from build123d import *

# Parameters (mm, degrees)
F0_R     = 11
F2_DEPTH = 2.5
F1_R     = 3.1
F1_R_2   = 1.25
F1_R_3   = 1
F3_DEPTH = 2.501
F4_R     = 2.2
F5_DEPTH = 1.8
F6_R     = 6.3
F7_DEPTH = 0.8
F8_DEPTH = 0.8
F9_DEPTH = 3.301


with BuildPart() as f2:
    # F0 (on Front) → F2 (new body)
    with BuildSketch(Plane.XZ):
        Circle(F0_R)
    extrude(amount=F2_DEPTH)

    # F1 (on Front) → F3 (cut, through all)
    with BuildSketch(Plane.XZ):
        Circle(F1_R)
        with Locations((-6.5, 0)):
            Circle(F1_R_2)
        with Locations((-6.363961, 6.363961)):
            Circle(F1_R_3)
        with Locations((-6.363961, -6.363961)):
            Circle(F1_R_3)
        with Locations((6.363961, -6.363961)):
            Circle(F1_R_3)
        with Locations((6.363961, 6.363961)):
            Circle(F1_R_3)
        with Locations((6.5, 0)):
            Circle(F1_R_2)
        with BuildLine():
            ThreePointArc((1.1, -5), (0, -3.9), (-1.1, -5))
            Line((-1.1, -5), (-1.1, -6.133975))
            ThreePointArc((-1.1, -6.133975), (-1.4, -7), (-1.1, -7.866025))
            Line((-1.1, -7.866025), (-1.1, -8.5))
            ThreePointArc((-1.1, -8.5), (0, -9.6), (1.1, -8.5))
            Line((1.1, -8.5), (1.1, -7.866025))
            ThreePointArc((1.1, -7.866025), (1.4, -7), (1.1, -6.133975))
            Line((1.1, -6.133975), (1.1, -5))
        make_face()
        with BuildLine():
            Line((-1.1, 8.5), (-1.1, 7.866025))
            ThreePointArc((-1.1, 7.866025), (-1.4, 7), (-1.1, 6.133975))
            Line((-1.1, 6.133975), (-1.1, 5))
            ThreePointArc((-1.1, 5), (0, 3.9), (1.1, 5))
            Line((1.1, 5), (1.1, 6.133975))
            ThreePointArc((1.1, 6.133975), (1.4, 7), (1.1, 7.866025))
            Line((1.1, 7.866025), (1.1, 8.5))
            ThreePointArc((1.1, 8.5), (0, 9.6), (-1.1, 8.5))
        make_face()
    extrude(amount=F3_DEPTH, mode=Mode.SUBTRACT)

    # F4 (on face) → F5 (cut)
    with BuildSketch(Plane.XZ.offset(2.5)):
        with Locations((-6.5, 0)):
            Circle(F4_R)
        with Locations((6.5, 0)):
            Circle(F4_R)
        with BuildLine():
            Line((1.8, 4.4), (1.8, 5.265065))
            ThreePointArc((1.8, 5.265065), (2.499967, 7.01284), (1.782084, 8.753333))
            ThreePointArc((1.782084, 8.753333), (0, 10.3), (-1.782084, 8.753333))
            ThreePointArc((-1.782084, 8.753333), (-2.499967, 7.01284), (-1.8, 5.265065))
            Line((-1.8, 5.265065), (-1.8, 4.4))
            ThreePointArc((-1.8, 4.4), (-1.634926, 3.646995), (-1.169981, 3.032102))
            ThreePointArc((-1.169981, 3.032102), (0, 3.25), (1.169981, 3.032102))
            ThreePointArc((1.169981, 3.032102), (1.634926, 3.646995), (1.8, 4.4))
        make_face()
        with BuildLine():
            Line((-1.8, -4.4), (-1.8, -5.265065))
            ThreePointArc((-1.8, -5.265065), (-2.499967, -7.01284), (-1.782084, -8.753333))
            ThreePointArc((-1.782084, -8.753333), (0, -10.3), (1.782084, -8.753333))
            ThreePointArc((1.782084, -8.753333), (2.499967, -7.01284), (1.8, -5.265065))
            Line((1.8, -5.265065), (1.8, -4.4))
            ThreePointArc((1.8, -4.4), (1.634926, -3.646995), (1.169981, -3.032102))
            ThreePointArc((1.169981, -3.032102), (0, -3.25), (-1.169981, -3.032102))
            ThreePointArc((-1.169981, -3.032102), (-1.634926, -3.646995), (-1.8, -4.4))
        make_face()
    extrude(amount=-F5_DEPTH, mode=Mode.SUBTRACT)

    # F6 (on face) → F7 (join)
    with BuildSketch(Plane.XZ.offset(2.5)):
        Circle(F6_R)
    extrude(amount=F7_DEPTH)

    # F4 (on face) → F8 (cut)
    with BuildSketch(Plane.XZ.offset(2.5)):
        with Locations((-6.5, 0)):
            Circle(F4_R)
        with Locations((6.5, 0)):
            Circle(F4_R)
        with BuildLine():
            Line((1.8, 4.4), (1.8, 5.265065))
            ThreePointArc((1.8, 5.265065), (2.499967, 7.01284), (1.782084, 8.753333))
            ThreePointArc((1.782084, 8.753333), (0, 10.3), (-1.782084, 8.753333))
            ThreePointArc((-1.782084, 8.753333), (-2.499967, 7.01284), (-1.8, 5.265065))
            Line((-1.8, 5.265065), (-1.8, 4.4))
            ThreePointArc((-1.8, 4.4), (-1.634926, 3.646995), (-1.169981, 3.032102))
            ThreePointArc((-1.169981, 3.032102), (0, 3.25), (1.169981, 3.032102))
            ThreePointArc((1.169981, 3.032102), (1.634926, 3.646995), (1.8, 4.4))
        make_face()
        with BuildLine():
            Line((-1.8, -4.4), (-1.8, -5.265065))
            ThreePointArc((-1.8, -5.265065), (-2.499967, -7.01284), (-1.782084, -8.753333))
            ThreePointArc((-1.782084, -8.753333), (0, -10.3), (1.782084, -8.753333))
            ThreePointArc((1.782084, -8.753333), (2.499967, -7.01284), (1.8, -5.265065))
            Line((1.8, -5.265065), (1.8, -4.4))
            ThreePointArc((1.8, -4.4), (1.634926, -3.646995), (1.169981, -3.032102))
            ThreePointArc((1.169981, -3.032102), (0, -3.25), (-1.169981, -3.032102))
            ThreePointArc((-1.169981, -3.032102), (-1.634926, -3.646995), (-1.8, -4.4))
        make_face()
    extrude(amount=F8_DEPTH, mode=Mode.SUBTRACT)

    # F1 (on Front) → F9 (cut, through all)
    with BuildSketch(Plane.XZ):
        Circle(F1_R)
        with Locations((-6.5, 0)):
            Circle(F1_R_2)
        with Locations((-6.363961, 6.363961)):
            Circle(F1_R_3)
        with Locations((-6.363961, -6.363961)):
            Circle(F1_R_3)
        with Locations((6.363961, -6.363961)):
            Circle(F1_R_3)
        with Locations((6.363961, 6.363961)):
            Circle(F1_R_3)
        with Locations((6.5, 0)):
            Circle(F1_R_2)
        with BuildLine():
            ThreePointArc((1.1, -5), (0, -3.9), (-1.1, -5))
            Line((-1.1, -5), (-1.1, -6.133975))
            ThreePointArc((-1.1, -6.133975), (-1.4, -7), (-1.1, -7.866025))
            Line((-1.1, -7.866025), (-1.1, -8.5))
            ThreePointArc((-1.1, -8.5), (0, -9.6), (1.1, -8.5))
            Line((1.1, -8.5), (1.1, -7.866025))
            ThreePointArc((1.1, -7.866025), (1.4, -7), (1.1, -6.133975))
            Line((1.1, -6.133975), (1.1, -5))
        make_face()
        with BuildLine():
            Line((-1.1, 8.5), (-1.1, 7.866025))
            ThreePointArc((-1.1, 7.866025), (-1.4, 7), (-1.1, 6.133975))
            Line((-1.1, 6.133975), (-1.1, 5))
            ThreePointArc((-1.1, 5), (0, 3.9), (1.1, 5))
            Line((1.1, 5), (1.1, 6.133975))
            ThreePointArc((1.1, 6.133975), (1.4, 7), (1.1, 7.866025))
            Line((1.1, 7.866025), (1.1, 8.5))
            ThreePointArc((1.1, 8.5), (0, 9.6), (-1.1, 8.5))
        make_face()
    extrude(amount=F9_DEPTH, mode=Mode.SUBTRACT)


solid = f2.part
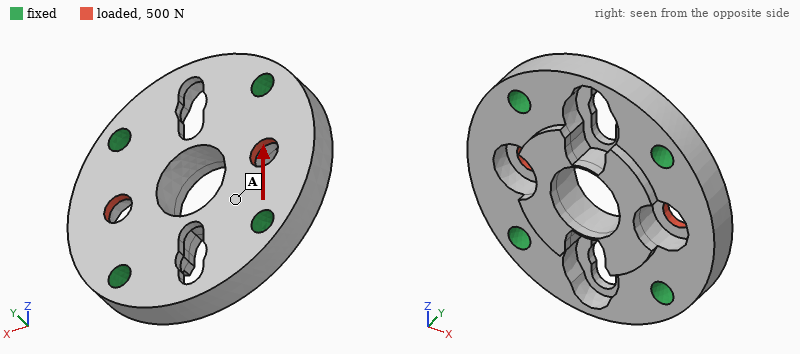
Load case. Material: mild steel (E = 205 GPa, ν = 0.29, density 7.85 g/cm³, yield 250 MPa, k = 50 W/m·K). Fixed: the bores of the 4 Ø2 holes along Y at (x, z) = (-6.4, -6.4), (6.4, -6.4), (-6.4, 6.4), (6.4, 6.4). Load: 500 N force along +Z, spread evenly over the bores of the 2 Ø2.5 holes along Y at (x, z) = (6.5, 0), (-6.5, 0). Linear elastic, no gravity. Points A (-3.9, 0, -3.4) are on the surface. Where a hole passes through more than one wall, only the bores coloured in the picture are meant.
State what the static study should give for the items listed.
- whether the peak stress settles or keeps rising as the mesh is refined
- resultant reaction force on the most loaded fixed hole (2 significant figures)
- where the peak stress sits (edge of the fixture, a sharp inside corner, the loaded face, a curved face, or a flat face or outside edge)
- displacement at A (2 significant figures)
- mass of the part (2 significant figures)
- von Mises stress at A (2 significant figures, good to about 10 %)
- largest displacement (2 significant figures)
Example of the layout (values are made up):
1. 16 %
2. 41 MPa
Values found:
1. keeps rising
2. 130 N
3. a sharp inside corner
4. 0.16 µm
5. 5.6 g
6. 8.4 MPa
7. 0.68 µm
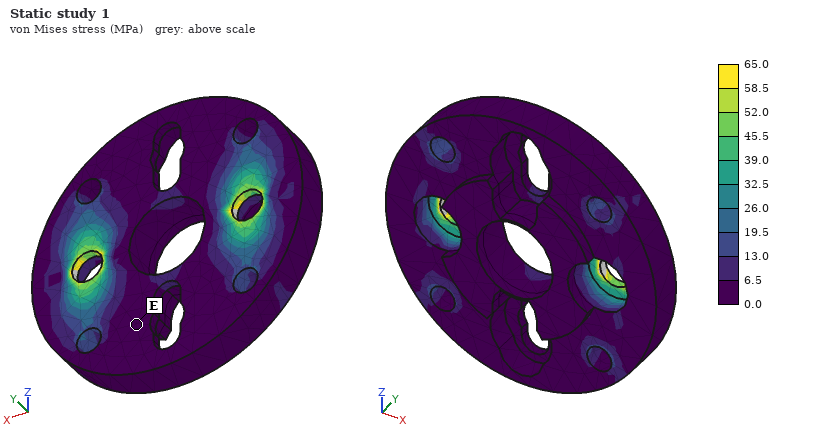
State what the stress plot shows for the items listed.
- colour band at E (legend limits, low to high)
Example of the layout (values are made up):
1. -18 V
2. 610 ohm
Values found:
1. 0.0 to 6.5 MPa
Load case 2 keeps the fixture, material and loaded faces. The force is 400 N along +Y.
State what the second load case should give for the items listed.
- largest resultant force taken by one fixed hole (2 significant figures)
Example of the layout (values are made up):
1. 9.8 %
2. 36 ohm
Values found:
1. 100 N
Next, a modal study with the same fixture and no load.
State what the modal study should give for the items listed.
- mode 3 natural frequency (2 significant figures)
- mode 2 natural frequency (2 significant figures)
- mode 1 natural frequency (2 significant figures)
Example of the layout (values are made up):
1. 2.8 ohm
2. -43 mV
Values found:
1. 62 kHz
2. 62 kHz
3. 60 kHz
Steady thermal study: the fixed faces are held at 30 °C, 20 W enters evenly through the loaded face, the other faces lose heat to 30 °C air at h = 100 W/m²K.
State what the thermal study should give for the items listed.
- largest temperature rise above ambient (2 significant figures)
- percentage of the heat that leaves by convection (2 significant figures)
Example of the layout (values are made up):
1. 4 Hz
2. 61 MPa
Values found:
1. 59 K
2. 6.0 %
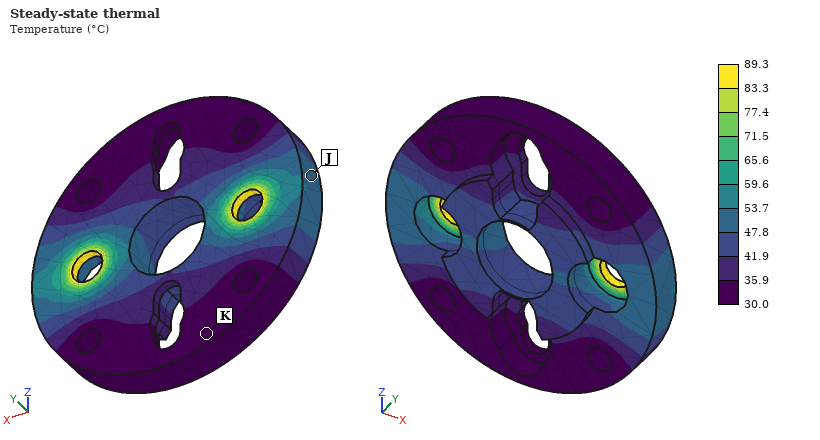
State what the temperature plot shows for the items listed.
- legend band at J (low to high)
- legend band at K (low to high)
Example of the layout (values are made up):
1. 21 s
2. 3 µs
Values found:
1. 47.8 to 53.7 °C
2. 30.0 to 35.9 °C
